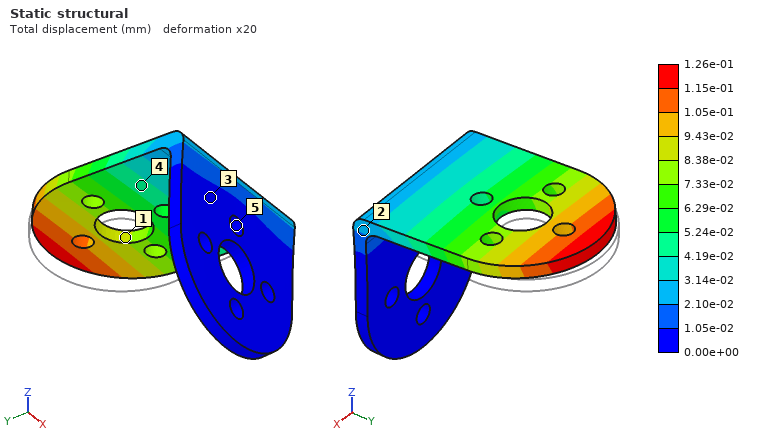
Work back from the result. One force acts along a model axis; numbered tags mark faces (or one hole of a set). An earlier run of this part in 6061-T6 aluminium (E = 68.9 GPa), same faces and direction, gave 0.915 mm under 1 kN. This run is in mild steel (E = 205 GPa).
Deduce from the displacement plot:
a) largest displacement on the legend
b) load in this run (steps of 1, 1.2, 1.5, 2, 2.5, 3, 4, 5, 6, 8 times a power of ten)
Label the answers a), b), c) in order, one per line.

a) 1.26e-01 mm
b) 400 N
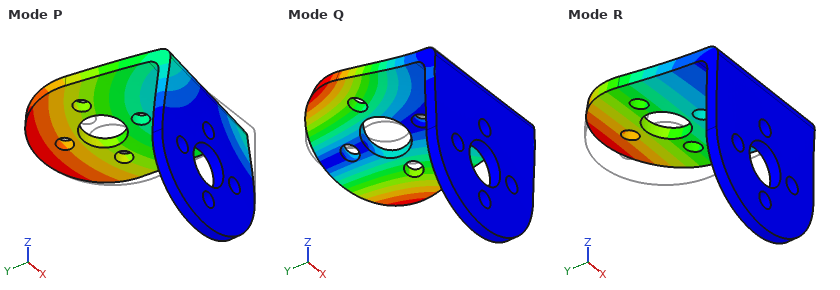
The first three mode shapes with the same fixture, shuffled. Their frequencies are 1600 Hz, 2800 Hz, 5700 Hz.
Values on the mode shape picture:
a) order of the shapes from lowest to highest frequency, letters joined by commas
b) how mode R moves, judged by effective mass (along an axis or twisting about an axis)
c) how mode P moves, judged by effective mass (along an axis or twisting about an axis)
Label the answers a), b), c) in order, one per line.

a) R, P, Q
b) along Z
c) along X
